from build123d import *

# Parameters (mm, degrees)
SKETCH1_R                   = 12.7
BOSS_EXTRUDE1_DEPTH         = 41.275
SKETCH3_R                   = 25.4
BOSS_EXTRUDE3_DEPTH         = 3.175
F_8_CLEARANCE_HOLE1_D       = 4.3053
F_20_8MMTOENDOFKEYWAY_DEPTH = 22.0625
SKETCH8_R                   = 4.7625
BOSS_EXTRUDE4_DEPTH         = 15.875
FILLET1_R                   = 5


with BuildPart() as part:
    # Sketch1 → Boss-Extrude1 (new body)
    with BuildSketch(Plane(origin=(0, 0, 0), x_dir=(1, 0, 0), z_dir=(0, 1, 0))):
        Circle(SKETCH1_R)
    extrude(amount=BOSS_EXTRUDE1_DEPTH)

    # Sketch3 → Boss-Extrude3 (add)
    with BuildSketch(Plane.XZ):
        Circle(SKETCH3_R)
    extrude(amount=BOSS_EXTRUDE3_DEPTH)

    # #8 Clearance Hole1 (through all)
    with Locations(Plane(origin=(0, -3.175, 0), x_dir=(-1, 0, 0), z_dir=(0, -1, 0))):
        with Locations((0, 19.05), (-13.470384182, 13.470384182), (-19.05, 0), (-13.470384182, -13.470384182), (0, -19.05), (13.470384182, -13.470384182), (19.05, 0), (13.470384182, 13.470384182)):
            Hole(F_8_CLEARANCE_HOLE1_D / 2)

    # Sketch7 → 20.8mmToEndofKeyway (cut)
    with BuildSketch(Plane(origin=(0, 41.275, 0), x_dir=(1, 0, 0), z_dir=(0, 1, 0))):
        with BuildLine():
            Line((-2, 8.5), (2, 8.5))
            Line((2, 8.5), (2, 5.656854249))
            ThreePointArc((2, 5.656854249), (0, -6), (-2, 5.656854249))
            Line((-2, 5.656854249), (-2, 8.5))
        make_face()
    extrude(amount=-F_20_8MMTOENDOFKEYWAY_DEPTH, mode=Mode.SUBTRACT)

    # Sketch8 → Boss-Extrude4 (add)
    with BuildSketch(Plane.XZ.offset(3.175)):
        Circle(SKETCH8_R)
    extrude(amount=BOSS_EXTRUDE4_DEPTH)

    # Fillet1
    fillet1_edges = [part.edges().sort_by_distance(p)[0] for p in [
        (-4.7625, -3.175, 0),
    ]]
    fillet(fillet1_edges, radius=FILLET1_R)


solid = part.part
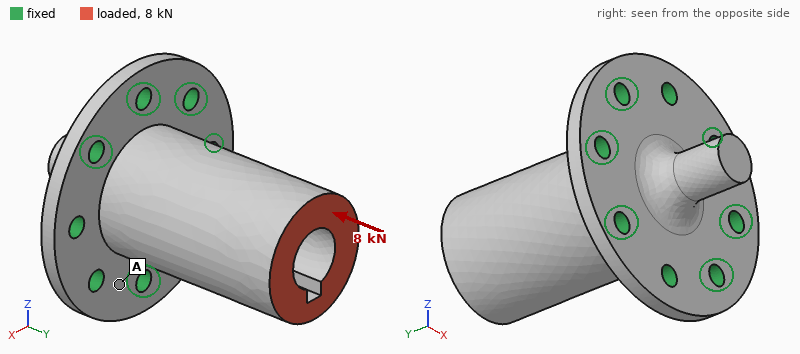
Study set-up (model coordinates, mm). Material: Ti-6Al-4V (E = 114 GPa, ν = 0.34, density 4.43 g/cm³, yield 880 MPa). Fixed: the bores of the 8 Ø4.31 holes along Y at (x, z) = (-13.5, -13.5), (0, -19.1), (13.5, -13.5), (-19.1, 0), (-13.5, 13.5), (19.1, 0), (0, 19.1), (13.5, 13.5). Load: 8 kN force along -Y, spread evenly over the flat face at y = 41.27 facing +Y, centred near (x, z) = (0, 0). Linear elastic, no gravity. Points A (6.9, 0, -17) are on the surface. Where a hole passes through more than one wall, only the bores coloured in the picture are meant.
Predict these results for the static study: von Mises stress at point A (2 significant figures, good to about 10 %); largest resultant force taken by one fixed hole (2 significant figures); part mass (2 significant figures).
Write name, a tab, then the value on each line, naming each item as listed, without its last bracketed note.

von Mises stress at point A	34 MPa
largest resultant force taken by one fixed hole	1.1 kN
part mass	110 g
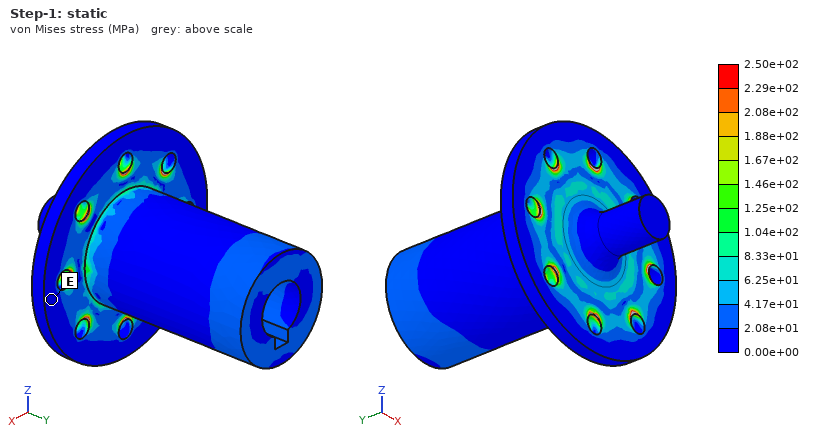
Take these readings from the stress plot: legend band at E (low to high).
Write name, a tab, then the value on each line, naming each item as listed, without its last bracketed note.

legend band at E	0.00e+00 to 2.08e+01 MPa
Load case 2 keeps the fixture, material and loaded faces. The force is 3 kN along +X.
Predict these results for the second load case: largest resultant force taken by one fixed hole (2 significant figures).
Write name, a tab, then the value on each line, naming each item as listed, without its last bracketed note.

largest resultant force taken by one fixed hole	2.2 kN
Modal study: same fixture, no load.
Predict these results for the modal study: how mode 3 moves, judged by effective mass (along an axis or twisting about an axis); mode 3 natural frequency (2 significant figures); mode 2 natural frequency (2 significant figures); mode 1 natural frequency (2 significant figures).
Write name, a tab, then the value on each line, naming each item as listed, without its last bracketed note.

how mode 3 moves, judged by effective mass	along Y
mode 3 natural frequency	12 kHz
mode 2 natural frequency	5200 Hz
mode 1 natural frequency	5200 Hz
